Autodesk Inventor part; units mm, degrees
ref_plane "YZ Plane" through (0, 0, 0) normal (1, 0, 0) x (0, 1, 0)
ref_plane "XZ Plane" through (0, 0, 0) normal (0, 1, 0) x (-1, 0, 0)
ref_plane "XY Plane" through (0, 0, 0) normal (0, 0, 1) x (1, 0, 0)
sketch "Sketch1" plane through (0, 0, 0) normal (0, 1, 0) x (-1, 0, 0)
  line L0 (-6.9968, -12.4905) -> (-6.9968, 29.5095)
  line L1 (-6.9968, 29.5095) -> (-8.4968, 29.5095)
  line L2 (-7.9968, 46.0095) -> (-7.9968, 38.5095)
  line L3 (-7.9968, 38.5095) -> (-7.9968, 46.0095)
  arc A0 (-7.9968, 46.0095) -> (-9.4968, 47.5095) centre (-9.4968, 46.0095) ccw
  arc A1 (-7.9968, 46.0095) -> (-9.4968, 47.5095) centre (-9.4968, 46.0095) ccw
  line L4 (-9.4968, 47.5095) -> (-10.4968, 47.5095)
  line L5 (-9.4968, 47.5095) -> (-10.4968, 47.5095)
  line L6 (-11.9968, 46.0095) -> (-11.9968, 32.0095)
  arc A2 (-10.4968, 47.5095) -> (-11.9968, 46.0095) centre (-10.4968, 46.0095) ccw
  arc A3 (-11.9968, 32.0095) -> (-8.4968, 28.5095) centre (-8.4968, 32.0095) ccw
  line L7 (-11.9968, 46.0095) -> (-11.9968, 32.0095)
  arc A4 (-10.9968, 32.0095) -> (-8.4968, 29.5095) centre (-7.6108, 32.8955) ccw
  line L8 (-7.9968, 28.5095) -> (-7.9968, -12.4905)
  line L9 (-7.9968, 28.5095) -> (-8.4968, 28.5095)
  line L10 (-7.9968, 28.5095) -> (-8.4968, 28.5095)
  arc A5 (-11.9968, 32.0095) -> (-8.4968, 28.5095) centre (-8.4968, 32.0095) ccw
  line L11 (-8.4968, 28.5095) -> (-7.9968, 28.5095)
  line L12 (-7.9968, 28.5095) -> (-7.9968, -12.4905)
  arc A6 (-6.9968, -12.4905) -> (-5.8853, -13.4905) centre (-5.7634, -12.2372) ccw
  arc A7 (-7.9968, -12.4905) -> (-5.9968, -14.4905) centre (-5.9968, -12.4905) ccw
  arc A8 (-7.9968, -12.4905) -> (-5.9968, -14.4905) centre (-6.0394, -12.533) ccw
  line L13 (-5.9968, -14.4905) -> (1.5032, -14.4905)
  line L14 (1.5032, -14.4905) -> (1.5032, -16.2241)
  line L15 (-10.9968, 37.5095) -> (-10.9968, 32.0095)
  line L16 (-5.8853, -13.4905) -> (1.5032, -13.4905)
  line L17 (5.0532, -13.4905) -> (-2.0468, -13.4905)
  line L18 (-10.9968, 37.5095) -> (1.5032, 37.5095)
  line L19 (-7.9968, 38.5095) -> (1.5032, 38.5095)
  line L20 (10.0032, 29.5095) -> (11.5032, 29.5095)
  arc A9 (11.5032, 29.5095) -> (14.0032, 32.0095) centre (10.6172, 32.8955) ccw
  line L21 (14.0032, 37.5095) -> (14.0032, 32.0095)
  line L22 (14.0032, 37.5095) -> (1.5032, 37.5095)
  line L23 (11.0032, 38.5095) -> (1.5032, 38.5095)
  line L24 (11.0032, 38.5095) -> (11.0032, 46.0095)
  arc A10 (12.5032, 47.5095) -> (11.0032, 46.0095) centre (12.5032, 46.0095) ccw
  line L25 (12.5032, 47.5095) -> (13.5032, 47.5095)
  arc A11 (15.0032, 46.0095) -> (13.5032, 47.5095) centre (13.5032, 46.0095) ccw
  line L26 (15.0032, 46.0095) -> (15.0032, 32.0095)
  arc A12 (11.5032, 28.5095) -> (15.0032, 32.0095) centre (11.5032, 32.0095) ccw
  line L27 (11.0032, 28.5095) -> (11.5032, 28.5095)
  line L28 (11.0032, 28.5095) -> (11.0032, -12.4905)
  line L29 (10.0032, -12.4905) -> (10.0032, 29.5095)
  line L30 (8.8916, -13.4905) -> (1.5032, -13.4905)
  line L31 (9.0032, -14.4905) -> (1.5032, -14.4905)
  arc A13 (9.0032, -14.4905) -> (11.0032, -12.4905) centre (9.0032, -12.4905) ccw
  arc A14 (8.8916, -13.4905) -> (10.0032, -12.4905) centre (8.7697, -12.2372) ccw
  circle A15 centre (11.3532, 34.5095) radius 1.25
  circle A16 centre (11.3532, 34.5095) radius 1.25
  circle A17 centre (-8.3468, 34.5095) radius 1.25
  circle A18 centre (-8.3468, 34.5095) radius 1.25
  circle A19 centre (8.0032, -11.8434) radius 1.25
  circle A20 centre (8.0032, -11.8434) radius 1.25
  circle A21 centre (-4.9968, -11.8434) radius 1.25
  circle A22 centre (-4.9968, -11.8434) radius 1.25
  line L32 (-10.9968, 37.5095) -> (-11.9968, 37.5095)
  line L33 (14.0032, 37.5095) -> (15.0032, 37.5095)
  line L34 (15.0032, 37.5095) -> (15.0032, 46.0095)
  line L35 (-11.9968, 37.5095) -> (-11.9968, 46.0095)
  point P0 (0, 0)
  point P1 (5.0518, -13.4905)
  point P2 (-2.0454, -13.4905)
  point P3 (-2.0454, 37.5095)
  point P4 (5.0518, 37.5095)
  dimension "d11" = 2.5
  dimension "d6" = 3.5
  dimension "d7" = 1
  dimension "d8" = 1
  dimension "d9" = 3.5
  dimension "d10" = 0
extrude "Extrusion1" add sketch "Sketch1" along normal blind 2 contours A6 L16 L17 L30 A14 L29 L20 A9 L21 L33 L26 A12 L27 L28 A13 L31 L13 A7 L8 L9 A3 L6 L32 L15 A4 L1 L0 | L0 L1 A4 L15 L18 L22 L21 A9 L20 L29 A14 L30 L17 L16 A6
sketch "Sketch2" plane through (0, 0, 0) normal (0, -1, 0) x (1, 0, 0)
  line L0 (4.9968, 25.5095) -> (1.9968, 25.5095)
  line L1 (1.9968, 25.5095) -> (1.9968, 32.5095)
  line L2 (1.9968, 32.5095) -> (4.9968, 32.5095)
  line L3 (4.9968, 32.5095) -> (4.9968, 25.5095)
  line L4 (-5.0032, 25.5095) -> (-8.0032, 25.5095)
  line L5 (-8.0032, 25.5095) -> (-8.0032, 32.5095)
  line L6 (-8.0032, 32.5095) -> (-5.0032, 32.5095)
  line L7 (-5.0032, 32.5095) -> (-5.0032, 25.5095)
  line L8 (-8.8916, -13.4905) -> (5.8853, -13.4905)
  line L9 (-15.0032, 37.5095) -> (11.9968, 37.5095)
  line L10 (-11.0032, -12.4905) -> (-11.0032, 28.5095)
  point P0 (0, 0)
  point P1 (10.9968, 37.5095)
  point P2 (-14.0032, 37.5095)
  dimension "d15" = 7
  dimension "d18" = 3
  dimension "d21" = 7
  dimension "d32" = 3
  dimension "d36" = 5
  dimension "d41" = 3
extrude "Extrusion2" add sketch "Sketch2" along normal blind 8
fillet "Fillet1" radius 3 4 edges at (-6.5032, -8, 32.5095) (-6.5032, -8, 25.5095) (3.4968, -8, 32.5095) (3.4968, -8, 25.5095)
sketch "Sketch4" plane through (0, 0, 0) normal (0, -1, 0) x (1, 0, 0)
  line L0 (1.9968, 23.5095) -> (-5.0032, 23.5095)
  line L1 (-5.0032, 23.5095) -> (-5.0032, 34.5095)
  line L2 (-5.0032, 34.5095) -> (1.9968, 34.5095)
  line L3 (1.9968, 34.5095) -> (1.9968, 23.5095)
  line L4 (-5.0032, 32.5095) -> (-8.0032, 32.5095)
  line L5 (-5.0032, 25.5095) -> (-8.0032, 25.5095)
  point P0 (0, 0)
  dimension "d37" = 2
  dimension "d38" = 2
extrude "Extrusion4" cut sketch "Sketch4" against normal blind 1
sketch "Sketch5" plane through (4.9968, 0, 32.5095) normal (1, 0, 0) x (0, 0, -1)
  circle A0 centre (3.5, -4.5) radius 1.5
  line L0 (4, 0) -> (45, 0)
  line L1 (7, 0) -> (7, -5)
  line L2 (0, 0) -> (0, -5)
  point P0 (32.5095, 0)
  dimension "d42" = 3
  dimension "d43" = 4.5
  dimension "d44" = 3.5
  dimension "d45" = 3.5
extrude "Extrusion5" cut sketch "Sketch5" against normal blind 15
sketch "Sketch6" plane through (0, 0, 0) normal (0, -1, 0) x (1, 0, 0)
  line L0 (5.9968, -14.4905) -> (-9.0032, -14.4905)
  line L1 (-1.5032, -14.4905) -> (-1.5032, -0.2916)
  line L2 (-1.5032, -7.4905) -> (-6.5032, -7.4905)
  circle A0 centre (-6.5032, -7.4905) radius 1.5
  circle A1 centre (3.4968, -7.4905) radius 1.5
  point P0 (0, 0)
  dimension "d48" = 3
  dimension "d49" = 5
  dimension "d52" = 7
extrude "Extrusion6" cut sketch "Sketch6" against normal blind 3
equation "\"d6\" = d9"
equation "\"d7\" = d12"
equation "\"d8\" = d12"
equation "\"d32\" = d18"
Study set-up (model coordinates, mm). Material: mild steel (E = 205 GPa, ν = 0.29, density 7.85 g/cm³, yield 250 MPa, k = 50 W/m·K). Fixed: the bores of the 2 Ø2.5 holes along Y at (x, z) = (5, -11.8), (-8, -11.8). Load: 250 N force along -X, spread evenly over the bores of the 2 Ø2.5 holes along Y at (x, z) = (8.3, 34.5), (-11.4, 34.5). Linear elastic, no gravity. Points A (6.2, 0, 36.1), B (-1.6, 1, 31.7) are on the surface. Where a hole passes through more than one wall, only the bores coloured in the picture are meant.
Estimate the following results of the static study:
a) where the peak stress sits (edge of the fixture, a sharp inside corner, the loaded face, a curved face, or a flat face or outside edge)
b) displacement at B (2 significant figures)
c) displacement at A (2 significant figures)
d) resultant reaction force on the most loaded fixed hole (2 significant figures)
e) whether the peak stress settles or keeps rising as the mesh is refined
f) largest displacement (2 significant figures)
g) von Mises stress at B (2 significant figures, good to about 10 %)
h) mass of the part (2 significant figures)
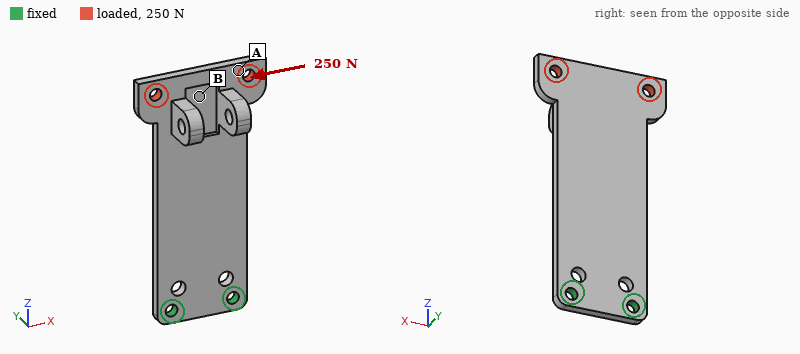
edge of the fixture
42 µm
49 µm
800 N
keeps rising
54 µm
33 MPa
18 g
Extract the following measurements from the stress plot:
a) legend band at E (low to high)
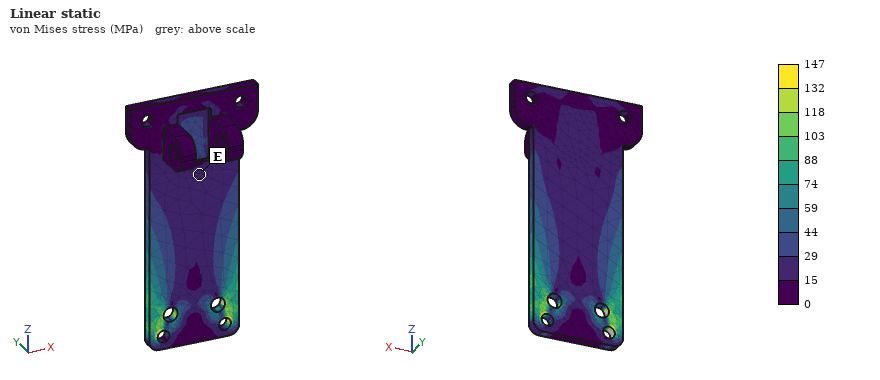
15 to 29 MPa
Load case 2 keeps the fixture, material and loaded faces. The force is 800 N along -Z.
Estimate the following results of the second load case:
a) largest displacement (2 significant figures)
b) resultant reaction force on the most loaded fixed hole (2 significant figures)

7.7 µm
410 N
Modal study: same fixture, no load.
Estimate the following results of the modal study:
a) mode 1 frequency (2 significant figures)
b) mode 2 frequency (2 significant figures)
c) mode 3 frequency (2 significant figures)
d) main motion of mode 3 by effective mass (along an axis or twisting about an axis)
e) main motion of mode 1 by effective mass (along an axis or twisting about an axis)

540 Hz
2400 Hz
3800 Hz
along Y
along Y
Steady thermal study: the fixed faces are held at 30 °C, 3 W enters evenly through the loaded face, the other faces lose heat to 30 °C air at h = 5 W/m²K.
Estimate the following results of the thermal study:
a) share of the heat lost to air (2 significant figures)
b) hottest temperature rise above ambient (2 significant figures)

18 %
72 K
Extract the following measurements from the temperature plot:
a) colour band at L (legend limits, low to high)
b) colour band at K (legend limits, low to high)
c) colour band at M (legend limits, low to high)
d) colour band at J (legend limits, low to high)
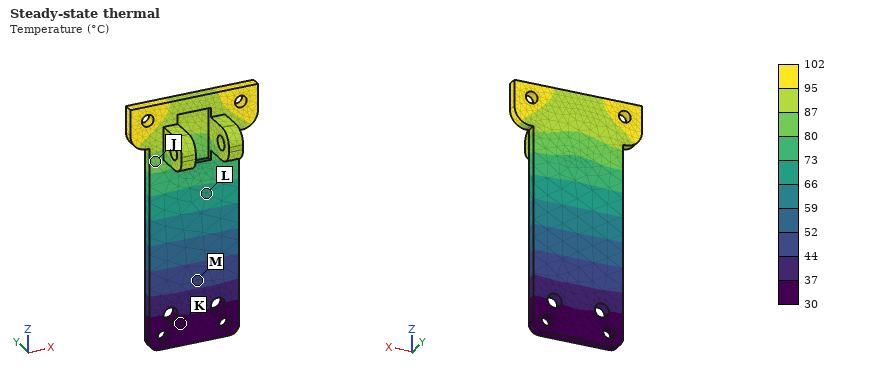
66 to 73 °C
30 to 37 °C
44 to 52 °C
80 to 87 °C
